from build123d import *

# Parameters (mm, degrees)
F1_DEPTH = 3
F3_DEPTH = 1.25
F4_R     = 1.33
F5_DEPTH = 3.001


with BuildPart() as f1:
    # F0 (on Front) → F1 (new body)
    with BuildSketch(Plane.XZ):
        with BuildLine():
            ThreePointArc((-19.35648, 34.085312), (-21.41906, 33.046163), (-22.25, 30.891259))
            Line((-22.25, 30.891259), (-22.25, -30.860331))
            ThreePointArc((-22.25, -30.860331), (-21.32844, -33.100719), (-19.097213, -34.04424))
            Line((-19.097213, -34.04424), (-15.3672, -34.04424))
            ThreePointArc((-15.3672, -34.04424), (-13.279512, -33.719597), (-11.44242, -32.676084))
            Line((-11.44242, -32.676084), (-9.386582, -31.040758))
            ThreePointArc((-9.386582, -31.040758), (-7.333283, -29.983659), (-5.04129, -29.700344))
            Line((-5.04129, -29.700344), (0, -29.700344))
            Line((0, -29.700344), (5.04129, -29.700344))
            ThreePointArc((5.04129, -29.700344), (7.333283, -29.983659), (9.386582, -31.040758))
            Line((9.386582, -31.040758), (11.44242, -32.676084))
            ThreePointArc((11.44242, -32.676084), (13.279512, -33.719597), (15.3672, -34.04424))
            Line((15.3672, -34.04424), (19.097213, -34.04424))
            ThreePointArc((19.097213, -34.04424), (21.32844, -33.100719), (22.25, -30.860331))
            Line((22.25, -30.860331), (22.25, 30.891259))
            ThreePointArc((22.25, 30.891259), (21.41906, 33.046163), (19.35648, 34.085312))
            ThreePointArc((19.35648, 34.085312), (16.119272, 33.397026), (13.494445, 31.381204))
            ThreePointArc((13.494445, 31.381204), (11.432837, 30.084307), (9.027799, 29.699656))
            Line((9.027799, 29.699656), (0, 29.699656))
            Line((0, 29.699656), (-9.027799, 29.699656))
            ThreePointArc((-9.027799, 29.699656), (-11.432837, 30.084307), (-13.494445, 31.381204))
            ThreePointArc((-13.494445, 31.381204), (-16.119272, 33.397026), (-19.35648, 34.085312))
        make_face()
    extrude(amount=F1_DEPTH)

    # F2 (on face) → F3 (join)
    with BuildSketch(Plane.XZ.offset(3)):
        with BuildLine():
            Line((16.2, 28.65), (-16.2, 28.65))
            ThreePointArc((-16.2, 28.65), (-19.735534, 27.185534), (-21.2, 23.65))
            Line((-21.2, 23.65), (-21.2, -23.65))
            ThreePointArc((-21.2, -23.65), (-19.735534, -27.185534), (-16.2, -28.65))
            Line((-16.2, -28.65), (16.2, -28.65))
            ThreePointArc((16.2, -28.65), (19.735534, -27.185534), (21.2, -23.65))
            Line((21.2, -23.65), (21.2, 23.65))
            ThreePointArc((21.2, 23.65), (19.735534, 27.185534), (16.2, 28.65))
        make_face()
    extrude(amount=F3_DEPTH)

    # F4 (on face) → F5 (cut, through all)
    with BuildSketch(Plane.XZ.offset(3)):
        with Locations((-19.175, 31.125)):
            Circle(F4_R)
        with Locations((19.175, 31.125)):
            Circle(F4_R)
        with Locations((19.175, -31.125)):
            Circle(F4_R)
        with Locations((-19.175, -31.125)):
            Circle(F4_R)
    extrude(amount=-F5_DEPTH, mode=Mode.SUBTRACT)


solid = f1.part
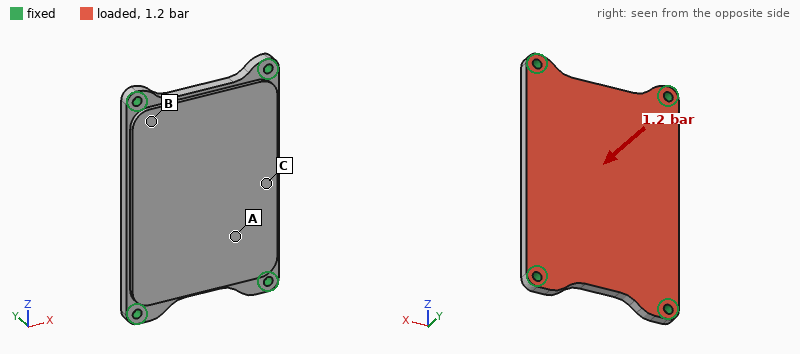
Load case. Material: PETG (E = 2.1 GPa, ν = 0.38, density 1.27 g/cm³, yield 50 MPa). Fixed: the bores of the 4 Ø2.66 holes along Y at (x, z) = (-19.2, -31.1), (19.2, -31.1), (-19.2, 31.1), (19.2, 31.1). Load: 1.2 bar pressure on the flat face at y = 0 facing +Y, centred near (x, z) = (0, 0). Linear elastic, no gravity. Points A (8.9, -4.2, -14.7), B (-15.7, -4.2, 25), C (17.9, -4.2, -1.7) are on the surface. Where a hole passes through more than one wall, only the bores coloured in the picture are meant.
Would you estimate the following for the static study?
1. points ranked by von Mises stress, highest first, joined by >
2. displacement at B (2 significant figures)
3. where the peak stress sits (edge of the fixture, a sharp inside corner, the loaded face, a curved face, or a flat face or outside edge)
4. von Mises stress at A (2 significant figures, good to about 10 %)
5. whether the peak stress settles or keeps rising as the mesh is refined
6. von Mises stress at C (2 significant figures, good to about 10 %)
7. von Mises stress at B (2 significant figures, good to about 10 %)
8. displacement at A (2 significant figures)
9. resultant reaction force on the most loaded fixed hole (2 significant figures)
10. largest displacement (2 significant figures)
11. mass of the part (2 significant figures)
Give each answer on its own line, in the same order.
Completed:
C > A > B
0.21 mm
edge of the fixture
6.8 MPa
keeps rising
12 MPa
3.7 MPa
0.58 mm
120 N
0.82 mm
14 g
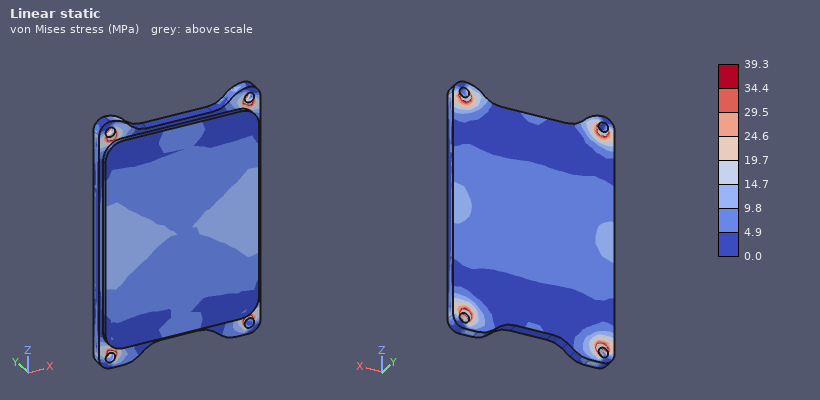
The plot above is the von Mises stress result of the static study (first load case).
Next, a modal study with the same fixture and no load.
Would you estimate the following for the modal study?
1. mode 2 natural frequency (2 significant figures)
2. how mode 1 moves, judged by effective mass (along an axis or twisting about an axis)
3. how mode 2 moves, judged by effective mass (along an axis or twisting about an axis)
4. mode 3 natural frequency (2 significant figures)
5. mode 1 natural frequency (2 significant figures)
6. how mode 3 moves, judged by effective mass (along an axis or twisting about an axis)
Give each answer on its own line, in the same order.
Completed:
1600 Hz
along Y
twisting about Z
2500 Hz
960 Hz
twisting about X
